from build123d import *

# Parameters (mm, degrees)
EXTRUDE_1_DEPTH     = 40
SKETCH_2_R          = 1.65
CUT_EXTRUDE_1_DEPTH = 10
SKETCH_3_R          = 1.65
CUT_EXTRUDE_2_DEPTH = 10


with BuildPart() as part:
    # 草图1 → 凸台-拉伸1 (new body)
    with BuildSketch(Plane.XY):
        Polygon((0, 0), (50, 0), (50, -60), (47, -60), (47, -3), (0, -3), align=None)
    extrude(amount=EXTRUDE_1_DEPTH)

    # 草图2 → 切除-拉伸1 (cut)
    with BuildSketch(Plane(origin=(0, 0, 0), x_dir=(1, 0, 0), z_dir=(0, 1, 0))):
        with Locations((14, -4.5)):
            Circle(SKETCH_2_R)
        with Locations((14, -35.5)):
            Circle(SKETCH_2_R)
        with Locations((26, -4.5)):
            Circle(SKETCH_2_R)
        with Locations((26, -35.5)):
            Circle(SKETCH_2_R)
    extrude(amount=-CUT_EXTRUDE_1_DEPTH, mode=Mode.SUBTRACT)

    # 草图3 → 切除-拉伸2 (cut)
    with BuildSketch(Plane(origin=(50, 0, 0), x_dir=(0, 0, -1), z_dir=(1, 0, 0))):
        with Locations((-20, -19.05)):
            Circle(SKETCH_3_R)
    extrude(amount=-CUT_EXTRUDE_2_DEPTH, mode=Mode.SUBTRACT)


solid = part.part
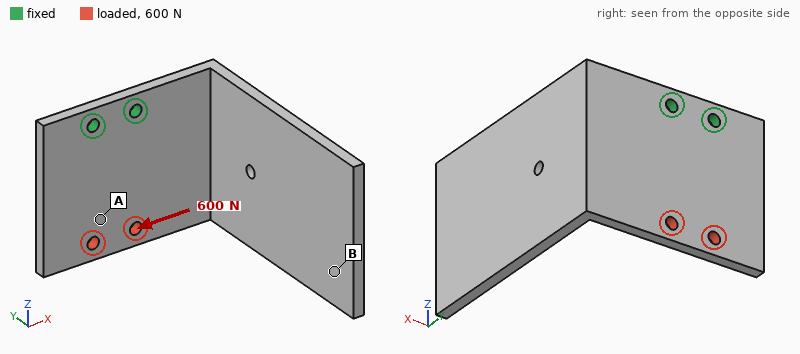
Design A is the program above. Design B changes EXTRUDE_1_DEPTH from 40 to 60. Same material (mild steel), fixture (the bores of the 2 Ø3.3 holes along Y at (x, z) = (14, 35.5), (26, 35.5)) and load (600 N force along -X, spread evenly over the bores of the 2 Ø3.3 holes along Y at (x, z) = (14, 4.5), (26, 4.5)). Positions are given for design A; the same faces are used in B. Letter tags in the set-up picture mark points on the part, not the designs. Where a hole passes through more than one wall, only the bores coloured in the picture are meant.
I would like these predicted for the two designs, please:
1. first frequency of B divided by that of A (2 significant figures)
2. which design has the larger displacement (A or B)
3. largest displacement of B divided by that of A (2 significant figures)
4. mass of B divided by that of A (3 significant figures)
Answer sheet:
1.1
A
0.70
1.51
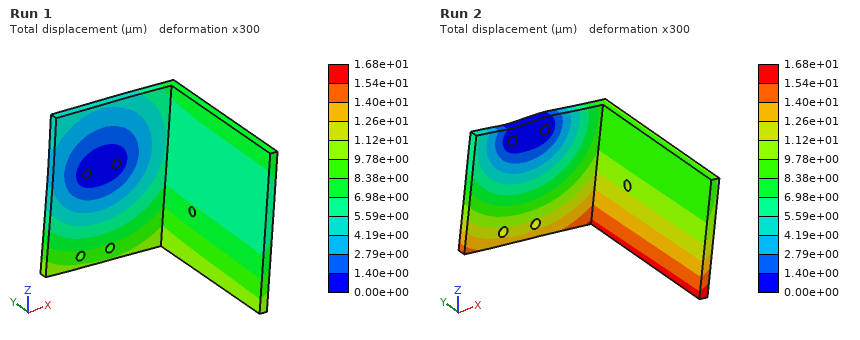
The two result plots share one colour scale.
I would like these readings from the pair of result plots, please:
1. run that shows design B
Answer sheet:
Run 1
